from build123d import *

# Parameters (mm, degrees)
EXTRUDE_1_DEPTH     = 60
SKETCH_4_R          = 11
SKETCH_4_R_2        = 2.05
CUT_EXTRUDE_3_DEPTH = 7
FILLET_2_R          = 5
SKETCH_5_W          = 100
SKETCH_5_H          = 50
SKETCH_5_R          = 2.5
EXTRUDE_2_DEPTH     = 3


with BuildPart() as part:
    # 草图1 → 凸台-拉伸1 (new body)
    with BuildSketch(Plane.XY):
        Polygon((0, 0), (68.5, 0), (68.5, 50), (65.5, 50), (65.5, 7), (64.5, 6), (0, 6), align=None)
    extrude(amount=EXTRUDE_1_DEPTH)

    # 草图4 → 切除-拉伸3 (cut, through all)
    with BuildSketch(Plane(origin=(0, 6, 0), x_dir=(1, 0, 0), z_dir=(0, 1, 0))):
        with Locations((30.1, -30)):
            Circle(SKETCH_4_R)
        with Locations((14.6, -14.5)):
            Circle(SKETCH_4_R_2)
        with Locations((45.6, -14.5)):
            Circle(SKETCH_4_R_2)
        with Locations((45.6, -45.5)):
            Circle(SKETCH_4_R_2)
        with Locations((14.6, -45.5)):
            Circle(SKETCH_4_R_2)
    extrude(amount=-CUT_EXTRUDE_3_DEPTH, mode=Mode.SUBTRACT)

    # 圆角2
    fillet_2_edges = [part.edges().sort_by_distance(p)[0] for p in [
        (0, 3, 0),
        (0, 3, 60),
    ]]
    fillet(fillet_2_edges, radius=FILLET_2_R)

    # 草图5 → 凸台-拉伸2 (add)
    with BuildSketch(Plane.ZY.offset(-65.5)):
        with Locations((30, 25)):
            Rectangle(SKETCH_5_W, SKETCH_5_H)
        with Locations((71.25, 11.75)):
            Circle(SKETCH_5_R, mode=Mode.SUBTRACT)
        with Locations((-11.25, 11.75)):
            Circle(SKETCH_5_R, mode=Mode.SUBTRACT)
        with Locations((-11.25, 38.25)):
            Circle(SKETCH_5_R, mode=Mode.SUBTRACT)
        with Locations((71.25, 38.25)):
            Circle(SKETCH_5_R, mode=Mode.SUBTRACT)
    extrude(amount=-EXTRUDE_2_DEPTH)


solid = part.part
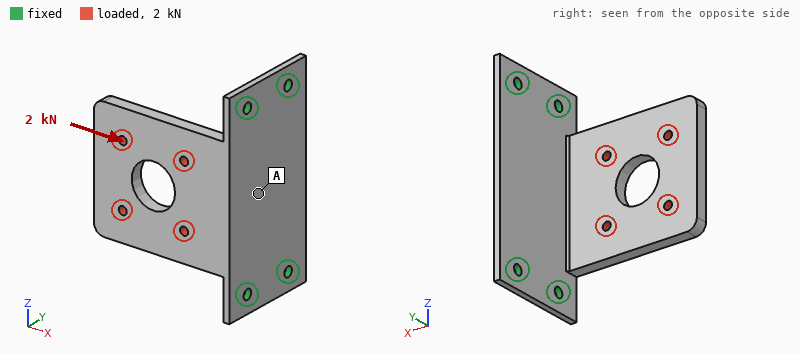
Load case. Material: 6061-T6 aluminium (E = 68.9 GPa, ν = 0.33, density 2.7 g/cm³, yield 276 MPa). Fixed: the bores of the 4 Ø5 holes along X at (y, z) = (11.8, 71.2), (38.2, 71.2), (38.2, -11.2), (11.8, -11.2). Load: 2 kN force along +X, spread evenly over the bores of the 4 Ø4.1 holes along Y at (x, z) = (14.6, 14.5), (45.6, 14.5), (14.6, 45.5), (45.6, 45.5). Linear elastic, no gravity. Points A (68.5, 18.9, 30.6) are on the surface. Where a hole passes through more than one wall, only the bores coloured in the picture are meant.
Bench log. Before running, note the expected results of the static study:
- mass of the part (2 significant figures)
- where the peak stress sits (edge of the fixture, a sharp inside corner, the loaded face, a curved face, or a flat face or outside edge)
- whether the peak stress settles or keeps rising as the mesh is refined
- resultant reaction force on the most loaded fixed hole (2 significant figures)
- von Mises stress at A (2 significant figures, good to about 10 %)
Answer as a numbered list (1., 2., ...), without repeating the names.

1. 96 g
2. edge of the fixture
3. keeps rising
4. 1.3 kN
5. 27 MPa
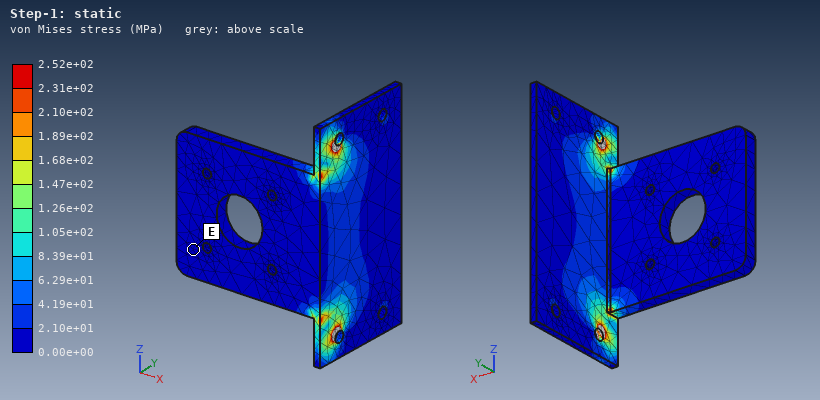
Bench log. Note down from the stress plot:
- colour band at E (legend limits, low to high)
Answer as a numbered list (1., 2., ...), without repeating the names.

1. 0.00e+00 to 2.10e+01 MPa
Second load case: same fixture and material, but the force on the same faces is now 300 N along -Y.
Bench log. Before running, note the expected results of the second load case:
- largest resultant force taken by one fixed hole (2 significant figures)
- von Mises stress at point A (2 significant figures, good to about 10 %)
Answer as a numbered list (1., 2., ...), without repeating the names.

1. 180 N
2. 40 MPa
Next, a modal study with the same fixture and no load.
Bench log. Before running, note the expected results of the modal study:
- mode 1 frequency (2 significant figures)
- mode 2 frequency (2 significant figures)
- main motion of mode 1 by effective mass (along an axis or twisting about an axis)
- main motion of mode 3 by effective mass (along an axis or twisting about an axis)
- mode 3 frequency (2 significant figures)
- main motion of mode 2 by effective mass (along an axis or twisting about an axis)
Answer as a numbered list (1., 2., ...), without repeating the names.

1. 500 Hz
2. 1900 Hz
3. along Y
4. along X
5. 2400 Hz
6. along Z
